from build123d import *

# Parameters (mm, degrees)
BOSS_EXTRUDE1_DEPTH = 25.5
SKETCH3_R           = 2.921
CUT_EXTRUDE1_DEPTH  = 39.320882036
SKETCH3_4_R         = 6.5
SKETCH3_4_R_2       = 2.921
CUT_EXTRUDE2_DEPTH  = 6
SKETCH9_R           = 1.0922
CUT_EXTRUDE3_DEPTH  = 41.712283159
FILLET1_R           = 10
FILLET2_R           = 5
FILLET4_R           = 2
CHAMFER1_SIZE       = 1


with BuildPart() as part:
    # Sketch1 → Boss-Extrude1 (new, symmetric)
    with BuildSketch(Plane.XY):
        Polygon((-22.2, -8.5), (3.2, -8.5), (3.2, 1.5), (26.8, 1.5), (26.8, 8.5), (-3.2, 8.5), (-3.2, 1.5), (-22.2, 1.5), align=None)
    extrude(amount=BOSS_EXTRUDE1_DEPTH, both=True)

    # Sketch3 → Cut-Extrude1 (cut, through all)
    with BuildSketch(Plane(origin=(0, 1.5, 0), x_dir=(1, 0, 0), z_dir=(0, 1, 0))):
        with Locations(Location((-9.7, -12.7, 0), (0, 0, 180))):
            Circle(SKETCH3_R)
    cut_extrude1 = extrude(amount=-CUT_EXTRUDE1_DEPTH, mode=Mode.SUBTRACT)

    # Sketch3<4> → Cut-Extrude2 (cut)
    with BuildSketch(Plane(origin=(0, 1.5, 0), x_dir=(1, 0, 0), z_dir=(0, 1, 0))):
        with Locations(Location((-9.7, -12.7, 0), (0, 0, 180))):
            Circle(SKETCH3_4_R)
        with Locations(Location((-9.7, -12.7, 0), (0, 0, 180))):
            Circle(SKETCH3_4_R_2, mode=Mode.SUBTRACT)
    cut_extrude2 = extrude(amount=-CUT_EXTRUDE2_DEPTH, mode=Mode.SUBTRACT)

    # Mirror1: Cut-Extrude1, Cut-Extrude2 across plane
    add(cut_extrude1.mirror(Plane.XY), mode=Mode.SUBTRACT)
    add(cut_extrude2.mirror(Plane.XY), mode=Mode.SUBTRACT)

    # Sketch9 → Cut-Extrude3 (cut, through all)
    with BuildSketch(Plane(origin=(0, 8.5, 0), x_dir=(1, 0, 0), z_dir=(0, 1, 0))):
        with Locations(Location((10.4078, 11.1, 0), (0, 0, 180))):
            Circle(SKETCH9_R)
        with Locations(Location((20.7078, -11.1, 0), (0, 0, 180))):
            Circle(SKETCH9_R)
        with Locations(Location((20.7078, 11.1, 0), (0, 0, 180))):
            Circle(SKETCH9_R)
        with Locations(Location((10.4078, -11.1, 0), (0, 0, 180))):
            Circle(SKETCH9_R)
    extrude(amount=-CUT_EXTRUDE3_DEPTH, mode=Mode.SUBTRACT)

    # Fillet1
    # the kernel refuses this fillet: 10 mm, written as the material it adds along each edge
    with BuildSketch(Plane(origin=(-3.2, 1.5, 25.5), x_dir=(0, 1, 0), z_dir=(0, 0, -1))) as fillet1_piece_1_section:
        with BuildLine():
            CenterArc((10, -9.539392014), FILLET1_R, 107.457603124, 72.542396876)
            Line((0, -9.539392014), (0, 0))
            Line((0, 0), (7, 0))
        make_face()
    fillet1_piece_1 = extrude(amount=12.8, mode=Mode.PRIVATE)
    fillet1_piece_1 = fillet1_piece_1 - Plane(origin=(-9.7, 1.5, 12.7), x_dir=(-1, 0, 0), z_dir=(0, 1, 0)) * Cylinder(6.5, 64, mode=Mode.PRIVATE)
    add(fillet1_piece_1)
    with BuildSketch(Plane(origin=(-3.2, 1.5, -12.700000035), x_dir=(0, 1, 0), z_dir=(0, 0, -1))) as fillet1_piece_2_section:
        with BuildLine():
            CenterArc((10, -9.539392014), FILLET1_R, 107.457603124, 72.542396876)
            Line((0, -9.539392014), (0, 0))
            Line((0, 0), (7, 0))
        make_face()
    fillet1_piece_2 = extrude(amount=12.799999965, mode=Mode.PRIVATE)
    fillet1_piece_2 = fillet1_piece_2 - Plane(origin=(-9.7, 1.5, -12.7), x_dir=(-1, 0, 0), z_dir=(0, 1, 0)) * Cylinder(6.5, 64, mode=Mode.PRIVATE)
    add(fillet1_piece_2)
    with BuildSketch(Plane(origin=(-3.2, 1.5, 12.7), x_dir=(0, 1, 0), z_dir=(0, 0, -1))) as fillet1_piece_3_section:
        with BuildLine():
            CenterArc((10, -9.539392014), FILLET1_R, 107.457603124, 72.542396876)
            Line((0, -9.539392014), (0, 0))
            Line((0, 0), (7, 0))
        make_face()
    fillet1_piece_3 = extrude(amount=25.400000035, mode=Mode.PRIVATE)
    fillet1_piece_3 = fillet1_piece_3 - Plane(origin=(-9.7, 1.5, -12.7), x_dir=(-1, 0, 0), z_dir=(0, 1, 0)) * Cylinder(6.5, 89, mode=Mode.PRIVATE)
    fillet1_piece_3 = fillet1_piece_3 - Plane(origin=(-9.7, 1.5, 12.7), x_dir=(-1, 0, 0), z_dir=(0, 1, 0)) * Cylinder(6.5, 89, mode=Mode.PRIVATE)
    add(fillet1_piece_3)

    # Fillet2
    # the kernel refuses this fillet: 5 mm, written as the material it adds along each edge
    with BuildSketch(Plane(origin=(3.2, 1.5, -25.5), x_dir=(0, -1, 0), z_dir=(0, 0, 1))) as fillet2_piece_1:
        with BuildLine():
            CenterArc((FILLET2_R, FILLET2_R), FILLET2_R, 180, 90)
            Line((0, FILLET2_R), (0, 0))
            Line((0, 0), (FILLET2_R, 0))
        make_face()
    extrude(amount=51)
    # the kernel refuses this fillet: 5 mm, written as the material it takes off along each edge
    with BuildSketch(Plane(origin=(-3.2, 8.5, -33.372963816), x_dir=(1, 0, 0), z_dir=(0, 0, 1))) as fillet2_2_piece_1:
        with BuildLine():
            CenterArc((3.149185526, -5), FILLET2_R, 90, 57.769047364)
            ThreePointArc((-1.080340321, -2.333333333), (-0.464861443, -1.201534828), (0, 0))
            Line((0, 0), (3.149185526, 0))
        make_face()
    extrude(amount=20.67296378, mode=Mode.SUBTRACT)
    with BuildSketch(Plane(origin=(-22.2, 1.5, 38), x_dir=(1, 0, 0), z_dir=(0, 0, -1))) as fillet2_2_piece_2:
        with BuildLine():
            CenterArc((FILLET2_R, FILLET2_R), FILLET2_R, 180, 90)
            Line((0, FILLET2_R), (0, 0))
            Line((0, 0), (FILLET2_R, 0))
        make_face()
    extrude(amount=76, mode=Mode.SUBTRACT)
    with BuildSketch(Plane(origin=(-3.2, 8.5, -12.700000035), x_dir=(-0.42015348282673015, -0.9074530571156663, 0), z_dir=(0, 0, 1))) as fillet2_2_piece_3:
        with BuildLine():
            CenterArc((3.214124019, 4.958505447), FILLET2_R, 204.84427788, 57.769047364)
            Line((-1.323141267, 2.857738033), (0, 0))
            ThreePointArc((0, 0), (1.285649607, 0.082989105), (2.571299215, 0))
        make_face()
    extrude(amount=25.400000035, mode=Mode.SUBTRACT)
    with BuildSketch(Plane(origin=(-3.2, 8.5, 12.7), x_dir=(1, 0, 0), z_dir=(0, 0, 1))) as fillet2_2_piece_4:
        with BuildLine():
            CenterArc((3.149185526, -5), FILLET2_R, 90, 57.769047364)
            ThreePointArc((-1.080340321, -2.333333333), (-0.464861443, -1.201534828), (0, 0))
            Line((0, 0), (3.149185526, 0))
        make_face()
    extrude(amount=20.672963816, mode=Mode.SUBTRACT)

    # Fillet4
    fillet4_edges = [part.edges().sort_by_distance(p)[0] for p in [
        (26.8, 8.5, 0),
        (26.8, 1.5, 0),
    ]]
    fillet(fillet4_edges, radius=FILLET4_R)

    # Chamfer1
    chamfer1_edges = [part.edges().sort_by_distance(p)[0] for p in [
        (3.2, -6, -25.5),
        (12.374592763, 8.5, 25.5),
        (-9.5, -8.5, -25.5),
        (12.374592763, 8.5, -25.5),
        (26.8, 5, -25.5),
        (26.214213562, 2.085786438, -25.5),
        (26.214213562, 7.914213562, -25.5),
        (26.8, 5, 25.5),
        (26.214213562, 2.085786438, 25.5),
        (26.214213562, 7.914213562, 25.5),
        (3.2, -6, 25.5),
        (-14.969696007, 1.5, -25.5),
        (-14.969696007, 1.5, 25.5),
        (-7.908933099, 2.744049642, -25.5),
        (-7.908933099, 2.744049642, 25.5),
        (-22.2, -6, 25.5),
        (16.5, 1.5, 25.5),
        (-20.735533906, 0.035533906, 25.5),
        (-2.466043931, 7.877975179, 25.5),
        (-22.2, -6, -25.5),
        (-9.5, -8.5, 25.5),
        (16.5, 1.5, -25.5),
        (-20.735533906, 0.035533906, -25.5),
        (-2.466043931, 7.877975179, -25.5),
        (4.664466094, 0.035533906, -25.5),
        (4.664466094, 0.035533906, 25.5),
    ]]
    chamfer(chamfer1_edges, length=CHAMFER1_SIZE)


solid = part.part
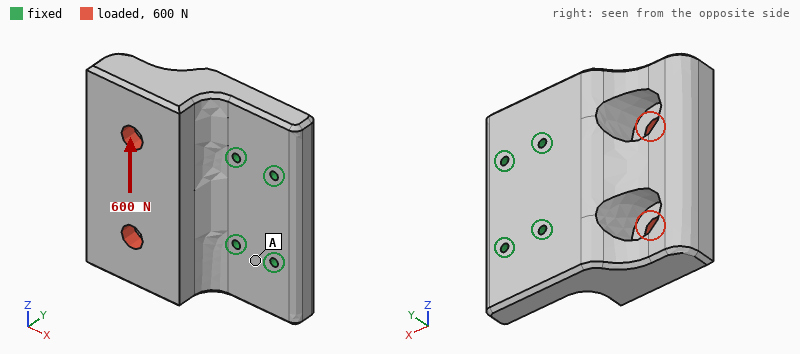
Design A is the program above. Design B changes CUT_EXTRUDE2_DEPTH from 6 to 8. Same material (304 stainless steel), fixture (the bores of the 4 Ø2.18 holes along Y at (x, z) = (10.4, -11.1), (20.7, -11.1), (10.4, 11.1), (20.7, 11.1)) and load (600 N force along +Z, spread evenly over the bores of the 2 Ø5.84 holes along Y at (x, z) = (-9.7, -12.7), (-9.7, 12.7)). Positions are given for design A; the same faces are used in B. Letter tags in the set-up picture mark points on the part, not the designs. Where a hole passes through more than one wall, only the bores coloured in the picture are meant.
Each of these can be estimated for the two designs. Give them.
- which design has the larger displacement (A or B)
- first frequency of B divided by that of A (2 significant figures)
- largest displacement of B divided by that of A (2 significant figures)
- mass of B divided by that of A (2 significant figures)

B
1.0
1.1
0.98
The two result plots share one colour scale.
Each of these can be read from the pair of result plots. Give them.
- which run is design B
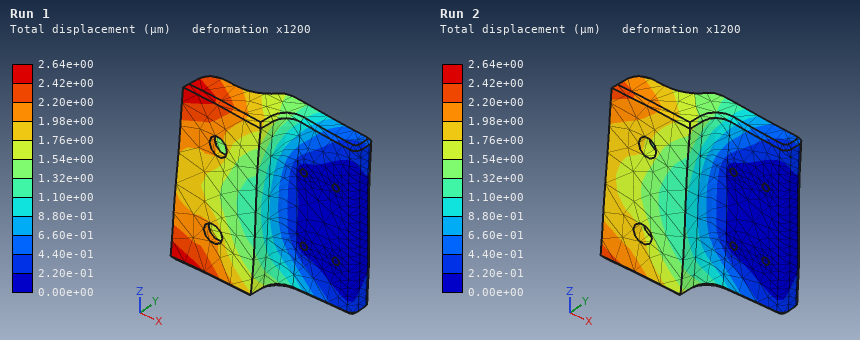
Run 1
